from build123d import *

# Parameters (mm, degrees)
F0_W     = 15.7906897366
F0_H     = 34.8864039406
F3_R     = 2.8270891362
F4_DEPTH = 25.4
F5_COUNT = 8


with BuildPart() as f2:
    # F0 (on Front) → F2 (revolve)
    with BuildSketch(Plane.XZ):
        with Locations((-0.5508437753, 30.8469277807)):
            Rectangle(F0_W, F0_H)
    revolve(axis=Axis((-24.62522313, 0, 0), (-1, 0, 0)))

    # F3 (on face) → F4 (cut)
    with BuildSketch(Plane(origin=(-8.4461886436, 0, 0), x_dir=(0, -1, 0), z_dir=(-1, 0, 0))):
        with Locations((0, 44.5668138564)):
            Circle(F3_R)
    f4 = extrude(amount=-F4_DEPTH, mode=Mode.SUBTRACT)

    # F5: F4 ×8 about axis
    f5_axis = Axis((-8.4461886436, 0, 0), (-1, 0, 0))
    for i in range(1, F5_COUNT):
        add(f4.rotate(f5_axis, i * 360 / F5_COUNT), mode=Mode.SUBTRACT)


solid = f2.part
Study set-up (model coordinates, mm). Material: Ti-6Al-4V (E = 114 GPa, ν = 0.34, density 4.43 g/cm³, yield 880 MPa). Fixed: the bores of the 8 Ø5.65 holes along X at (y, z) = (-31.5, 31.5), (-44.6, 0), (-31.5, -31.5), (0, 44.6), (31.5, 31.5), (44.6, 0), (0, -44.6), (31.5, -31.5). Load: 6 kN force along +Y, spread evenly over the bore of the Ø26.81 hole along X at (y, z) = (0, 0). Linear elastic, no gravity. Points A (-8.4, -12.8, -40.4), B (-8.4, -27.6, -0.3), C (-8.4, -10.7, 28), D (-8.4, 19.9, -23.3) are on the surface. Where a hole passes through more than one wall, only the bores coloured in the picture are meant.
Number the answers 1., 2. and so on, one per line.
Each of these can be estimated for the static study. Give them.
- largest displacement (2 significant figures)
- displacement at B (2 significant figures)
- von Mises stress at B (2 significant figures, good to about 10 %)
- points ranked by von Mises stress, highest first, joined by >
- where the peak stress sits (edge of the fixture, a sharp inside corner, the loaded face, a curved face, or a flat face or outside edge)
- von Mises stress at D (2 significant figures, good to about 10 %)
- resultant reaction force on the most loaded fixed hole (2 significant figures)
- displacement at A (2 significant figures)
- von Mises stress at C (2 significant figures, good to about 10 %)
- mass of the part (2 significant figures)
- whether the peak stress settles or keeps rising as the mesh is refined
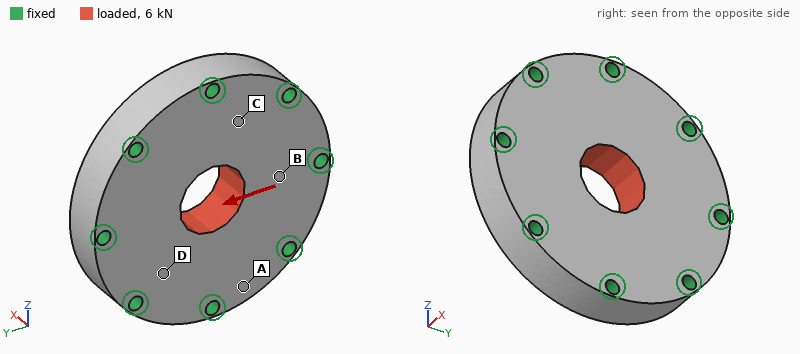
1. 1.2 µm
2. 0.68 µm
3. 4.3 MPa
4. B > D > C > A
5. edge of the fixture
6. 3.3 MPa
7. 1.2 kN
8. 0.19 µm
9. 1.7 MPa
10. 460 g
11. keeps rising
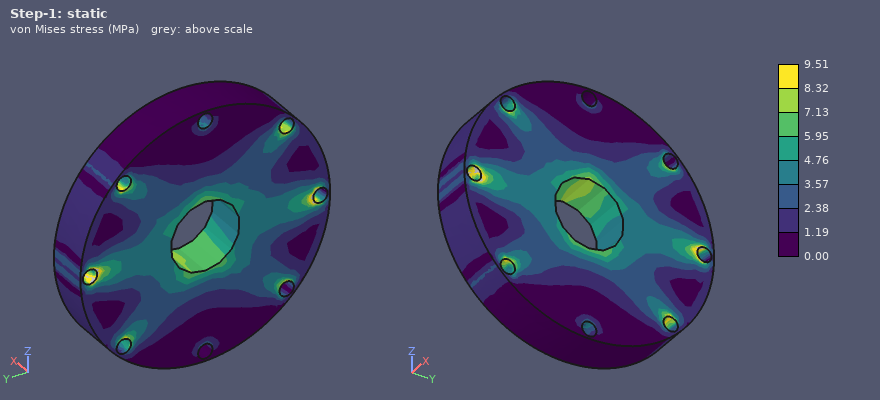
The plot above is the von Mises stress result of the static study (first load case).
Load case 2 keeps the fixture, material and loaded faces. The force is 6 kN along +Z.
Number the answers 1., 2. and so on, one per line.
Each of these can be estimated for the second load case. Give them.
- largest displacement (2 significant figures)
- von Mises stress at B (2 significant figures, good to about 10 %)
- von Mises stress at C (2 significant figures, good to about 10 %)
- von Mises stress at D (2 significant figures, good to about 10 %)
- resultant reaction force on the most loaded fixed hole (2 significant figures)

1. 1.2 µm
2. 1.3 MPa
3. 2.3 MPa
4. 3.1 MPa
5. 1.2 kN
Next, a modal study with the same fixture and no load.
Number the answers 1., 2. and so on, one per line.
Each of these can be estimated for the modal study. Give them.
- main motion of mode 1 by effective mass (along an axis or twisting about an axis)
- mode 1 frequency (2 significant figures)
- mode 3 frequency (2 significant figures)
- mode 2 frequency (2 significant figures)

1. along X
2. 14 kHz
3. 22 kHz
4. 22 kHz
